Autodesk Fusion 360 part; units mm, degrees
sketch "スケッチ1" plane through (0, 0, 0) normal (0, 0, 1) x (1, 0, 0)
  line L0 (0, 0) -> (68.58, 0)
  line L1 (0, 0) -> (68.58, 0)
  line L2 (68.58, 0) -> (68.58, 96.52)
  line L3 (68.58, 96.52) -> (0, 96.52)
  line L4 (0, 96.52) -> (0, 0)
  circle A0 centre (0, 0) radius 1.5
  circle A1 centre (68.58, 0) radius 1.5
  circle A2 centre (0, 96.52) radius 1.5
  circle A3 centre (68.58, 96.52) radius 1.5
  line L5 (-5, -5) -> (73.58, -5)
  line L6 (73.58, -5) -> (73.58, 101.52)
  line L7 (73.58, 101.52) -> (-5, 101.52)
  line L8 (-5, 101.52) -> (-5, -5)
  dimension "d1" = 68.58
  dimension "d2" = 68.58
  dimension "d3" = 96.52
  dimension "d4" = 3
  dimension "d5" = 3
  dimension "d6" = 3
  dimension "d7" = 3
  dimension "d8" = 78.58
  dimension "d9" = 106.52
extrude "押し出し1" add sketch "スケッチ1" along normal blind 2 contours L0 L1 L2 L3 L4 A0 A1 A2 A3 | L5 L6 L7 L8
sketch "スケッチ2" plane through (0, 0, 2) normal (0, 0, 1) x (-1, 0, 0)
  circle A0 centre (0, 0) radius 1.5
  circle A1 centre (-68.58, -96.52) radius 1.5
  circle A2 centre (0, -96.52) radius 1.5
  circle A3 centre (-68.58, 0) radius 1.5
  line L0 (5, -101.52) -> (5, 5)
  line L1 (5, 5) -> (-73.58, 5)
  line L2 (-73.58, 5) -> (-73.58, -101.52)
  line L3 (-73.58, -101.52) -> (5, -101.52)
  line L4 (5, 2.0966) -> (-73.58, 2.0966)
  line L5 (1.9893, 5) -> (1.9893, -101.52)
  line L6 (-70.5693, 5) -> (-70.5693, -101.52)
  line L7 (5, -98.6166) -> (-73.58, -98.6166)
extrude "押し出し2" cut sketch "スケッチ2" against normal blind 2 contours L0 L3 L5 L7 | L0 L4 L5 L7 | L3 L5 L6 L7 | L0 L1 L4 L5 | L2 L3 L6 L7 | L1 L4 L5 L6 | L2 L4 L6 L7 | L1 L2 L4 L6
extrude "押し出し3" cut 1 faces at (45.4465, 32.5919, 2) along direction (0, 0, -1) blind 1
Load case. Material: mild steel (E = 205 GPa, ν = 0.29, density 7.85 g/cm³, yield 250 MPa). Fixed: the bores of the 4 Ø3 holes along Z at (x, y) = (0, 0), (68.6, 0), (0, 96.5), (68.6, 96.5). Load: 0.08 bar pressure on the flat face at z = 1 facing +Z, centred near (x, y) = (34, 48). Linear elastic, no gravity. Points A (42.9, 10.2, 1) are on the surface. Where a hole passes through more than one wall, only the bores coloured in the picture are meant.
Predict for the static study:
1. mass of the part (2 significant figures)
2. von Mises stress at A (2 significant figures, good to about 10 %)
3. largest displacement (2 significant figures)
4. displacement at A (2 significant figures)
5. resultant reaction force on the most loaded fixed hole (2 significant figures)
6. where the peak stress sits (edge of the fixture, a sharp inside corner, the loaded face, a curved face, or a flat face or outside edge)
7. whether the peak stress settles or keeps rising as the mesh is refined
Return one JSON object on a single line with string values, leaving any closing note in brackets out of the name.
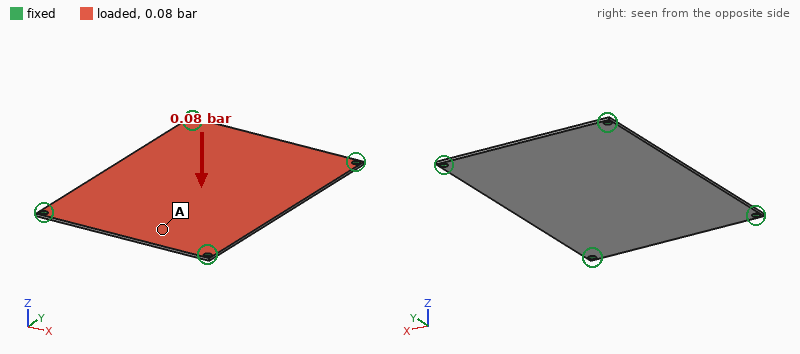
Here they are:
{"mass of the part": "57 g", "von Mises stress at A": "14 MPa", "largest displacement": "0.21 mm", "displacement at A": "0.087 mm", "resultant reaction force on the most loaded fixed hole": "15 N", "where the peak stress sits": "edge of the fixture", "whether the peak stress settles or keeps rising as the mesh is refined": "keeps rising"}
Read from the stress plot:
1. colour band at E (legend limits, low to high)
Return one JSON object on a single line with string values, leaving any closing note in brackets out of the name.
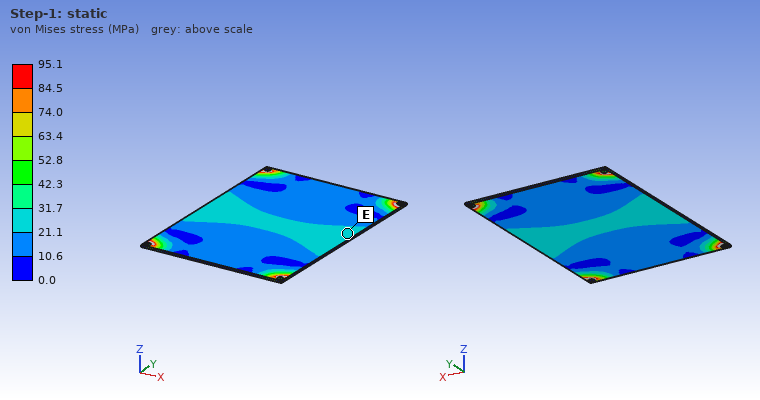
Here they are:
{"colour band at E": "21.1 to 31.7 MPa"}
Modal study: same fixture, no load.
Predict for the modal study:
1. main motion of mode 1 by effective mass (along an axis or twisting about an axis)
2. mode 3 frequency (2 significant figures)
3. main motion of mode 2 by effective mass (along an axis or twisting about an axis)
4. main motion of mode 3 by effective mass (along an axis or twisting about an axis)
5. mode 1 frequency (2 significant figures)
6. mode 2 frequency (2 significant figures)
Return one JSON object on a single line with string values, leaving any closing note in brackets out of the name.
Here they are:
{"main motion of mode 1 by effective mass": "along Z", "mode 3 frequency": "980 Hz", "main motion of mode 2 by effective mass": "twisting about Y", "main motion of mode 3 by effective mass": "twisting about X", "mode 1 frequency": "410 Hz", "mode 2 frequency": "730 Hz"}
